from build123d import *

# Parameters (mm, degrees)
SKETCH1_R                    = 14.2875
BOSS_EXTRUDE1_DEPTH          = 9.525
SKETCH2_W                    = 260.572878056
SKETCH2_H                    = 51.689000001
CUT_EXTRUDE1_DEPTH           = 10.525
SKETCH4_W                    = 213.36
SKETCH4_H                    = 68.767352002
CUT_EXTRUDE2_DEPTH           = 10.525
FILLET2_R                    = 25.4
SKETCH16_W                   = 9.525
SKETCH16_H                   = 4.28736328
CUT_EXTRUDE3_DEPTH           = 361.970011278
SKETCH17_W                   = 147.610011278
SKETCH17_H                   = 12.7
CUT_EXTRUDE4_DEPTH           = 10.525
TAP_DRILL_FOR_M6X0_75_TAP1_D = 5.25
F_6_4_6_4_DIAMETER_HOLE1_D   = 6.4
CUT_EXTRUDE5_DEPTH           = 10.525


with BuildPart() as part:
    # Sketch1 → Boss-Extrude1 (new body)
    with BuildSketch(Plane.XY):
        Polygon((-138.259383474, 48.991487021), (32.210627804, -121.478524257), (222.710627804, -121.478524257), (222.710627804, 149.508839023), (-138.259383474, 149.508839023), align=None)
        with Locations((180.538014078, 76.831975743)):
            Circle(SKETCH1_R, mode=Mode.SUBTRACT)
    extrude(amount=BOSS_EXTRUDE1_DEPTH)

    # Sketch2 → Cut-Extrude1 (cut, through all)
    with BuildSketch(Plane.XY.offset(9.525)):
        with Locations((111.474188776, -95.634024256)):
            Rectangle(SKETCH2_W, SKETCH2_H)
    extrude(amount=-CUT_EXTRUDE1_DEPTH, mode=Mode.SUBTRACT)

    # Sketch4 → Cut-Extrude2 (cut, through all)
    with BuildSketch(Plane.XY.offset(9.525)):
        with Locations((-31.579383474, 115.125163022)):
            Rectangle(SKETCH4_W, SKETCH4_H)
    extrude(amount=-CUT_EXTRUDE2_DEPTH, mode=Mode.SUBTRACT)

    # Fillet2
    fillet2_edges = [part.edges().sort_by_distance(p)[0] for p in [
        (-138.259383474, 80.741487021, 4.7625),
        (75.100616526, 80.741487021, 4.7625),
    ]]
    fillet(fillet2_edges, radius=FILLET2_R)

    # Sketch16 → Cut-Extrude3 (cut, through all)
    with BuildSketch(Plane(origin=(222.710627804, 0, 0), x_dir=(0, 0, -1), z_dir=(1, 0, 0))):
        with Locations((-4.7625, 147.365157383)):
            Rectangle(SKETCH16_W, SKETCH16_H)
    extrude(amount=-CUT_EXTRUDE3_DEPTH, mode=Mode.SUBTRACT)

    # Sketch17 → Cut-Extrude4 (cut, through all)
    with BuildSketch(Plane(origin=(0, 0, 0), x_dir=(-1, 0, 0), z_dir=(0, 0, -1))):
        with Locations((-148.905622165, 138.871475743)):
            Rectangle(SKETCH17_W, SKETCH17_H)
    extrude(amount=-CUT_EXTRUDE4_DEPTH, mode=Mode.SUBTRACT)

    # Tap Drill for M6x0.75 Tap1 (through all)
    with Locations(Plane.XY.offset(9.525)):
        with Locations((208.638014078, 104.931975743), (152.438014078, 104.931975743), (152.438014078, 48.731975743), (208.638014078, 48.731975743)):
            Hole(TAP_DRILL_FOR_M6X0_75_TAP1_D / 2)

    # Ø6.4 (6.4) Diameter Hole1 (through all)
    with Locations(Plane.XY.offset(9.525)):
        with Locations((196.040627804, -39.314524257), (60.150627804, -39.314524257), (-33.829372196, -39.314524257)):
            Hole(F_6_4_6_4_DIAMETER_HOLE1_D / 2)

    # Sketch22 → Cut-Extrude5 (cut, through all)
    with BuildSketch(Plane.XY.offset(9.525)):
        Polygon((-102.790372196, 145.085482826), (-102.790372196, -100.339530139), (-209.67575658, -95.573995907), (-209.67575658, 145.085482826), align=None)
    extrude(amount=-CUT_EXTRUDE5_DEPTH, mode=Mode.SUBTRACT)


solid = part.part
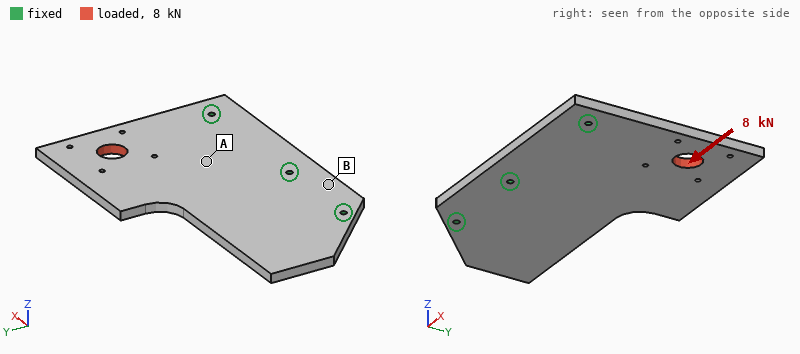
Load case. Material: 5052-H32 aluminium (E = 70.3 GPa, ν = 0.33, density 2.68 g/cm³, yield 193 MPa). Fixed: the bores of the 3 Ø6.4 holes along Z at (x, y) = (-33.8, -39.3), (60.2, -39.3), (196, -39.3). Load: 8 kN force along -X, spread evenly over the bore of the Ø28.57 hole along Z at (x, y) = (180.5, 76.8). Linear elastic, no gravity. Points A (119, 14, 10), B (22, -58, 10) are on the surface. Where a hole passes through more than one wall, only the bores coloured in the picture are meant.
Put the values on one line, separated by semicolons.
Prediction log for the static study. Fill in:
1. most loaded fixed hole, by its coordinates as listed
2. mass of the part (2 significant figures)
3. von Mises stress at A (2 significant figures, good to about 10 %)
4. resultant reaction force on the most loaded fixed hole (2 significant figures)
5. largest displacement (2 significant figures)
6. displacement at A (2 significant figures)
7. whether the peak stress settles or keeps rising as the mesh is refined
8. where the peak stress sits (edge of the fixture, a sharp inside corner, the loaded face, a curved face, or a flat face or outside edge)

(196, -39.3); 1.3 kg; 7.0 MPa; 5.3 kN; 40 µm; 12 µm; keeps rising; edge of the fixture
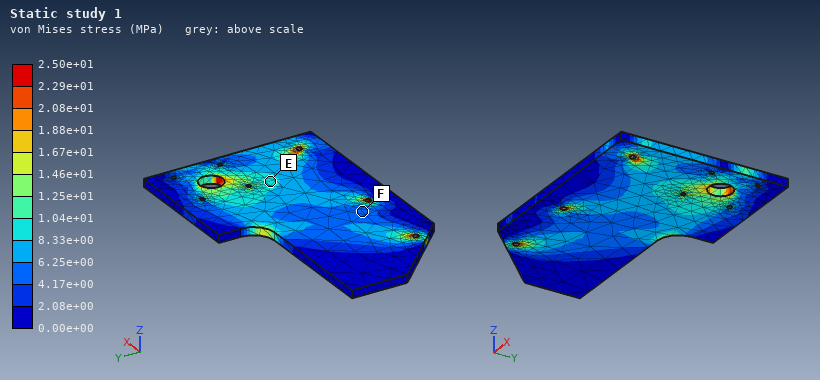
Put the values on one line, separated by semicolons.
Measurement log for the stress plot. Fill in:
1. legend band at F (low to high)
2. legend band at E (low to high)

4.17e+00 to 6.25e+00 MPa; 8.33e+00 to 1.04e+01 MPa
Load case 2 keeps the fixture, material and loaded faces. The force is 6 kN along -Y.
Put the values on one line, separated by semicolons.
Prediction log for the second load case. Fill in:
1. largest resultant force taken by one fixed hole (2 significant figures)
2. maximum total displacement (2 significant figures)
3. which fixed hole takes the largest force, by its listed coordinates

5.0 kN; 21 µm; (196, -39.3)
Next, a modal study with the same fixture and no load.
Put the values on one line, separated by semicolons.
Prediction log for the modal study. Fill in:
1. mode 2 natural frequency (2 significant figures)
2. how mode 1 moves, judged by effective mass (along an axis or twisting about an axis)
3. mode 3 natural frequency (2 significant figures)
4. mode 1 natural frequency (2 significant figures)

490 Hz; along Z; 810 Hz; 270 Hz
